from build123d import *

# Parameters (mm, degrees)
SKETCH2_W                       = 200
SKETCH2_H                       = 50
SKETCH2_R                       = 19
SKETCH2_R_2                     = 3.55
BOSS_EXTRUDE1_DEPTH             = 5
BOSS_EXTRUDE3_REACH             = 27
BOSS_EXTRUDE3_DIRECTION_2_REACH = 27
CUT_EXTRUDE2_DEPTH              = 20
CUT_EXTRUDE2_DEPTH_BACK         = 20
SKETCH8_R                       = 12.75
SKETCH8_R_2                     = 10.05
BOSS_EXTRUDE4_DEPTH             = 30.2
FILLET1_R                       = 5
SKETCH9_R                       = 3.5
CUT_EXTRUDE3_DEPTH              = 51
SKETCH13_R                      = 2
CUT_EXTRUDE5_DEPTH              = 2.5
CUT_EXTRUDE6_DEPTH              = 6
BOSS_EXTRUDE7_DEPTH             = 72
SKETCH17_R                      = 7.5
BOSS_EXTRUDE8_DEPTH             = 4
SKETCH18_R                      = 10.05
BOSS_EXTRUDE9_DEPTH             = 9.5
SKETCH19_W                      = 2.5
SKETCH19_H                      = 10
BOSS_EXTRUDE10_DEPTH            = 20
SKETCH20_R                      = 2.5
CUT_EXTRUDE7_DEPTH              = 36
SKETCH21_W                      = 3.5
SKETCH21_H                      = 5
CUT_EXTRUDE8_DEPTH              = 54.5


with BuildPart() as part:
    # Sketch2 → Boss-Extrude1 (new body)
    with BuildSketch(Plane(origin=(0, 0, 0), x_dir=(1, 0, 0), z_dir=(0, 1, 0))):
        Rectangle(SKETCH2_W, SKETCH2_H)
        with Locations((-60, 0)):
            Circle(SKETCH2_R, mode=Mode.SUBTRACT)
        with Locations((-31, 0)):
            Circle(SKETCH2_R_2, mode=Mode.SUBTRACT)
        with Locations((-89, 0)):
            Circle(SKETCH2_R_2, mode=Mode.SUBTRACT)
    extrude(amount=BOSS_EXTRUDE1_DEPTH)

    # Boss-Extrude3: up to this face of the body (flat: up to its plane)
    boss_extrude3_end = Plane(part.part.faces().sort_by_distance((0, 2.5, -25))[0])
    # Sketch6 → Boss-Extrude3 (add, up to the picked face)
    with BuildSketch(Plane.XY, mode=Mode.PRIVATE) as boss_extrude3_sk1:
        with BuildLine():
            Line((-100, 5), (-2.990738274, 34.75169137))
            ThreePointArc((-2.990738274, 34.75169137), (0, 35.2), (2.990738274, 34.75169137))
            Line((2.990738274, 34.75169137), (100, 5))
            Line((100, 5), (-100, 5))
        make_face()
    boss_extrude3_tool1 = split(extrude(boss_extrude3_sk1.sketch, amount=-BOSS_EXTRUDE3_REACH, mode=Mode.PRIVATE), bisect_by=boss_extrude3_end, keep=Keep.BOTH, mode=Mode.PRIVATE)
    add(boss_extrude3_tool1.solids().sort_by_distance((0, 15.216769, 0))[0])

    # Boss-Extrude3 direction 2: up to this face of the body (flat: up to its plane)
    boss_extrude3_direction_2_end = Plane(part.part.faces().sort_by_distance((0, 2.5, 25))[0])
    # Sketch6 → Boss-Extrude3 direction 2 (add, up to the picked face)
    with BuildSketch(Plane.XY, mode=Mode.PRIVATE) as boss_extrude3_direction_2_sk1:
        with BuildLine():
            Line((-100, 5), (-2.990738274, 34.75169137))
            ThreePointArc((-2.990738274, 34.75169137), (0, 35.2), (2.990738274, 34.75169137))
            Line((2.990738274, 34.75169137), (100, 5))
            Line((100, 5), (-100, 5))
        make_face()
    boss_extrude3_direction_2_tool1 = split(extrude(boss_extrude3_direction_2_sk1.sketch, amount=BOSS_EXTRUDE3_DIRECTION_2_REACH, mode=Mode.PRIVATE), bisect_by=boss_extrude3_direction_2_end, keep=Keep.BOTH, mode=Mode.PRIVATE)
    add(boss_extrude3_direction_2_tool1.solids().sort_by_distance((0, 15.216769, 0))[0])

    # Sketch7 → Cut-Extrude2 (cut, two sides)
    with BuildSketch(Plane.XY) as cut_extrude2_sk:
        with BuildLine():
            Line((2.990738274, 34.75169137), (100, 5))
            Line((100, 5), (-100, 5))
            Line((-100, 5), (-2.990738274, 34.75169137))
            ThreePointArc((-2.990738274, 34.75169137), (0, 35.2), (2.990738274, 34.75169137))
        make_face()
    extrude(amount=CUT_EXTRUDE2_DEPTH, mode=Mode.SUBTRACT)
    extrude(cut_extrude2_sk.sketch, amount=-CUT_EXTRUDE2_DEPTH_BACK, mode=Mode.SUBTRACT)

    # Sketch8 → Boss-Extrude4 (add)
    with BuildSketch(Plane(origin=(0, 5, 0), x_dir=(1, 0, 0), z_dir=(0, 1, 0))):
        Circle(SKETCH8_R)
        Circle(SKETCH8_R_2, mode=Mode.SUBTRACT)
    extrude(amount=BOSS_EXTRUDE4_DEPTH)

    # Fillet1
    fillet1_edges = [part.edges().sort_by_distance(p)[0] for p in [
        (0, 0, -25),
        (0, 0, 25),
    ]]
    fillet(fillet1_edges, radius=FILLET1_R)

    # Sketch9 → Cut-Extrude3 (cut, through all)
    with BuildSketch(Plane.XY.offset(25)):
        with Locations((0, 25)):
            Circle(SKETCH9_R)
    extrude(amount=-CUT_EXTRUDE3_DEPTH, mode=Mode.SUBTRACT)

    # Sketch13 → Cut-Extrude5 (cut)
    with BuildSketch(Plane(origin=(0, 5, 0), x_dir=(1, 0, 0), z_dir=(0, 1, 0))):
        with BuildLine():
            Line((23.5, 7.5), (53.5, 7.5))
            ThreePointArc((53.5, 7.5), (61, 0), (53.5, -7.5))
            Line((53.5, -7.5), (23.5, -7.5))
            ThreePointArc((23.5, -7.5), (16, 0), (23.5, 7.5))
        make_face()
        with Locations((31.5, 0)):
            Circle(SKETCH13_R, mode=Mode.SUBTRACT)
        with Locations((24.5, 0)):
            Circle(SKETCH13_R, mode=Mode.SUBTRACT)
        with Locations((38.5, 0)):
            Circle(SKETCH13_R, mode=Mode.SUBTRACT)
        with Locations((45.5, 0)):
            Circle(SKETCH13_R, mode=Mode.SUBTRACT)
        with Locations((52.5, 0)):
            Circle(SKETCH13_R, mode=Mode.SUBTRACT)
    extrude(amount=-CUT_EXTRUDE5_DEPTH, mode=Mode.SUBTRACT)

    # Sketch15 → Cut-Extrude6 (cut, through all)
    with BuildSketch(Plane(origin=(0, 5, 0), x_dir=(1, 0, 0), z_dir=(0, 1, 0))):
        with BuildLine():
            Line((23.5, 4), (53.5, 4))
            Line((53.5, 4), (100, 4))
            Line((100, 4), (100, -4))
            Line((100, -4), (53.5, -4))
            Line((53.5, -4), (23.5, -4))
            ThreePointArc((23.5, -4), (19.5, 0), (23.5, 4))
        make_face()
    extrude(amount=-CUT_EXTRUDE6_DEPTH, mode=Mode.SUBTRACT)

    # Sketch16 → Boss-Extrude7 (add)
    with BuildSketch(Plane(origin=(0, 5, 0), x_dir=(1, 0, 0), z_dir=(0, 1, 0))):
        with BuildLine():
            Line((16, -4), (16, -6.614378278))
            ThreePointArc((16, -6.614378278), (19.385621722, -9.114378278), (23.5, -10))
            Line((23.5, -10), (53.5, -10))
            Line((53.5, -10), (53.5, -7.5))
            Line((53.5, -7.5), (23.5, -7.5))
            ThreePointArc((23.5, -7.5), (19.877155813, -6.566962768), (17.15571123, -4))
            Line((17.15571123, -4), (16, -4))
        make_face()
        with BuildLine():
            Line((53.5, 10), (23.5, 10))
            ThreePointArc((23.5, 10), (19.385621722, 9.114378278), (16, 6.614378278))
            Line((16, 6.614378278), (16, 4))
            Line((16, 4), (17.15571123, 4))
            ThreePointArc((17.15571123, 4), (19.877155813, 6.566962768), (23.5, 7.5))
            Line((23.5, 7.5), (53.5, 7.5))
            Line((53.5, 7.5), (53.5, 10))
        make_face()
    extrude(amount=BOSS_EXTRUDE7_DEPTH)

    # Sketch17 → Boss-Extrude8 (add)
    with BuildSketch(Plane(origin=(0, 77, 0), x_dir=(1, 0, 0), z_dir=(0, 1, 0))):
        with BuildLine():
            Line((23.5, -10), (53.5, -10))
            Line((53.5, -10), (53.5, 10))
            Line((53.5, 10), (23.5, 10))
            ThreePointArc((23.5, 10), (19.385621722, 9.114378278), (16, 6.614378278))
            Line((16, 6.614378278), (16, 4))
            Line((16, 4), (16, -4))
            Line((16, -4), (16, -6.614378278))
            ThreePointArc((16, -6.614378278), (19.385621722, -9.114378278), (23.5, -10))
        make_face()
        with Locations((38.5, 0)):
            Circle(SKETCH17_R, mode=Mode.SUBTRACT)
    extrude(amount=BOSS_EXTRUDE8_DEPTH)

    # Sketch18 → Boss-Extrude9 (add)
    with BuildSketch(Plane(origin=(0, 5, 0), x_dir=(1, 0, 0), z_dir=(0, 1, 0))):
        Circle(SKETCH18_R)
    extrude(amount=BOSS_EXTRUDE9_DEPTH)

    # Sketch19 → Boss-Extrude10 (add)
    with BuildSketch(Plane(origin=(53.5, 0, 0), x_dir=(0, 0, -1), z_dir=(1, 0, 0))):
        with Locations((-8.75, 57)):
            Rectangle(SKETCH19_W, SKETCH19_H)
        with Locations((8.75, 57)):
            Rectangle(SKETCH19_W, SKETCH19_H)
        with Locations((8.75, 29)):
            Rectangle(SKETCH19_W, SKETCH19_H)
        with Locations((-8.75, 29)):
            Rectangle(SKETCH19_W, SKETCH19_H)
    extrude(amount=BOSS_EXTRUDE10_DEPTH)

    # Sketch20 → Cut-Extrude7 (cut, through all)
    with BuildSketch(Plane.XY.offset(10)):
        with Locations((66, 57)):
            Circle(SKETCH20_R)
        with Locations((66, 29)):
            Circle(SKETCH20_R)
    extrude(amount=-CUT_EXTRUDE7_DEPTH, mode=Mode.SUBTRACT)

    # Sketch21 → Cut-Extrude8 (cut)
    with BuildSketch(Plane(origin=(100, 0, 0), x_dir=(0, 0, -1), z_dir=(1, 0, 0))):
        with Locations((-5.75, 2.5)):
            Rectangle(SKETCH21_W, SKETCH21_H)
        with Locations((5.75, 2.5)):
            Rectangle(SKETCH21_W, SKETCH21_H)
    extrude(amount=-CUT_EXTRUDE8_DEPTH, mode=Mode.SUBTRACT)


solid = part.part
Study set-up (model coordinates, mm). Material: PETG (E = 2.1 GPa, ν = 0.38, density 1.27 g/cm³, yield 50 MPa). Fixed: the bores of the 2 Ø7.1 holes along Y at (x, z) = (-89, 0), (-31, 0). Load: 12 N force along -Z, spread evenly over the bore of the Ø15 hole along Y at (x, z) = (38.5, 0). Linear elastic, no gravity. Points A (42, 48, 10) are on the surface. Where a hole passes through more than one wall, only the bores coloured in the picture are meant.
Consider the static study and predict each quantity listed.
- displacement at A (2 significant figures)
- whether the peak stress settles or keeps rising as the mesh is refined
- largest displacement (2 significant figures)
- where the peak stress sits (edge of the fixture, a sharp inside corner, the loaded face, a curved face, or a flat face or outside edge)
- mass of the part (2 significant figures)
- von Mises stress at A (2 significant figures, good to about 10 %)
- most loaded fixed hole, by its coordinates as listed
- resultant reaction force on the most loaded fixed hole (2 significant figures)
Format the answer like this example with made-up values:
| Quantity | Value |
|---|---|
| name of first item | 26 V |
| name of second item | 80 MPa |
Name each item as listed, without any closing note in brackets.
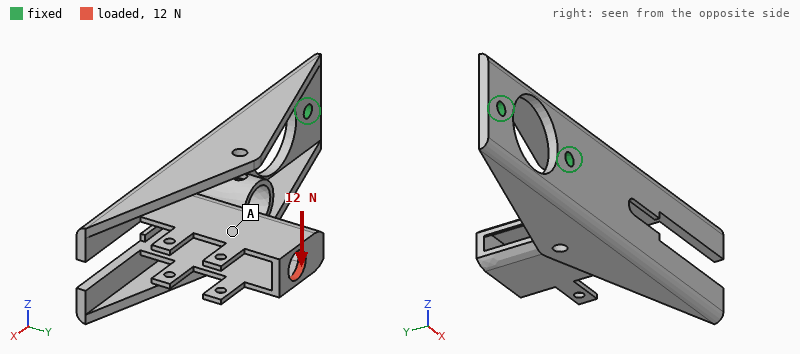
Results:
| Quantity | Value |
|---|---|
| displacement at A | 1.5 mm |
| whether the peak stress settles or keeps rising as the mesh is refined | keeps rising |
| largest displacement | 2.5 mm |
| where the peak stress sits | edge of the fixture |
| mass of the part | 120 g |
| von Mises stress at A | 0.77 MPa |
| most loaded fixed hole, by its coordinates as listed | (-31, 0) |
| resultant reaction force on the most loaded fixed hole | 18 N |
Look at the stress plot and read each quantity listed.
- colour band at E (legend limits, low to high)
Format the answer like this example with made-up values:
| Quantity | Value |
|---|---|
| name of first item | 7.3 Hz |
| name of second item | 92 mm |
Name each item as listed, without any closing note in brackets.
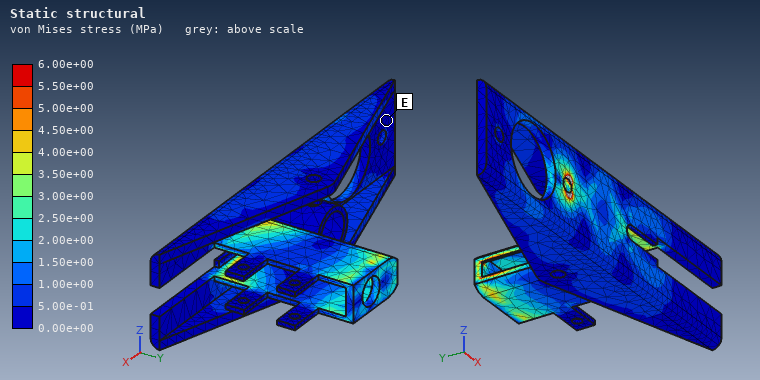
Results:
| Quantity | Value |
|---|---|
| colour band at E | 0.00e+00 to 5.00e-01 MPa |
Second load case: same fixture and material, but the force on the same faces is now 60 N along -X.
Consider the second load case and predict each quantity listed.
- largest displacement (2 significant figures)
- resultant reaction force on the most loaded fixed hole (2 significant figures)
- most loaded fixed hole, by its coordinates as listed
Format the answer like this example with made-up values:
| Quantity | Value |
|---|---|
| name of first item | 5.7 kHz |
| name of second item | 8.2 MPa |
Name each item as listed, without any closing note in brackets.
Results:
| Quantity | Value |
|---|---|
| largest displacement | 2.3 mm |
| resultant reaction force on the most loaded fixed hole | 110 N |
| most loaded fixed hole, by its coordinates as listed | (-89, 0) |
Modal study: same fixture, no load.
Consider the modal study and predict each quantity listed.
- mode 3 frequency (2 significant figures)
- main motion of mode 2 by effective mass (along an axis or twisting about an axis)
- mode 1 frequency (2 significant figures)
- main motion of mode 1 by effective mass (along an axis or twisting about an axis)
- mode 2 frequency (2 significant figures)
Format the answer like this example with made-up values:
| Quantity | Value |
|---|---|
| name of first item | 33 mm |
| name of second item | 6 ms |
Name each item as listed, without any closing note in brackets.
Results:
| Quantity | Value |
|---|---|
| mode 3 frequency | 250 Hz |
| main motion of mode 2 by effective mass | along Y |
| mode 1 frequency | 110 Hz |
| main motion of mode 1 by effective mass | along Z |
| mode 2 frequency | 160 Hz |
